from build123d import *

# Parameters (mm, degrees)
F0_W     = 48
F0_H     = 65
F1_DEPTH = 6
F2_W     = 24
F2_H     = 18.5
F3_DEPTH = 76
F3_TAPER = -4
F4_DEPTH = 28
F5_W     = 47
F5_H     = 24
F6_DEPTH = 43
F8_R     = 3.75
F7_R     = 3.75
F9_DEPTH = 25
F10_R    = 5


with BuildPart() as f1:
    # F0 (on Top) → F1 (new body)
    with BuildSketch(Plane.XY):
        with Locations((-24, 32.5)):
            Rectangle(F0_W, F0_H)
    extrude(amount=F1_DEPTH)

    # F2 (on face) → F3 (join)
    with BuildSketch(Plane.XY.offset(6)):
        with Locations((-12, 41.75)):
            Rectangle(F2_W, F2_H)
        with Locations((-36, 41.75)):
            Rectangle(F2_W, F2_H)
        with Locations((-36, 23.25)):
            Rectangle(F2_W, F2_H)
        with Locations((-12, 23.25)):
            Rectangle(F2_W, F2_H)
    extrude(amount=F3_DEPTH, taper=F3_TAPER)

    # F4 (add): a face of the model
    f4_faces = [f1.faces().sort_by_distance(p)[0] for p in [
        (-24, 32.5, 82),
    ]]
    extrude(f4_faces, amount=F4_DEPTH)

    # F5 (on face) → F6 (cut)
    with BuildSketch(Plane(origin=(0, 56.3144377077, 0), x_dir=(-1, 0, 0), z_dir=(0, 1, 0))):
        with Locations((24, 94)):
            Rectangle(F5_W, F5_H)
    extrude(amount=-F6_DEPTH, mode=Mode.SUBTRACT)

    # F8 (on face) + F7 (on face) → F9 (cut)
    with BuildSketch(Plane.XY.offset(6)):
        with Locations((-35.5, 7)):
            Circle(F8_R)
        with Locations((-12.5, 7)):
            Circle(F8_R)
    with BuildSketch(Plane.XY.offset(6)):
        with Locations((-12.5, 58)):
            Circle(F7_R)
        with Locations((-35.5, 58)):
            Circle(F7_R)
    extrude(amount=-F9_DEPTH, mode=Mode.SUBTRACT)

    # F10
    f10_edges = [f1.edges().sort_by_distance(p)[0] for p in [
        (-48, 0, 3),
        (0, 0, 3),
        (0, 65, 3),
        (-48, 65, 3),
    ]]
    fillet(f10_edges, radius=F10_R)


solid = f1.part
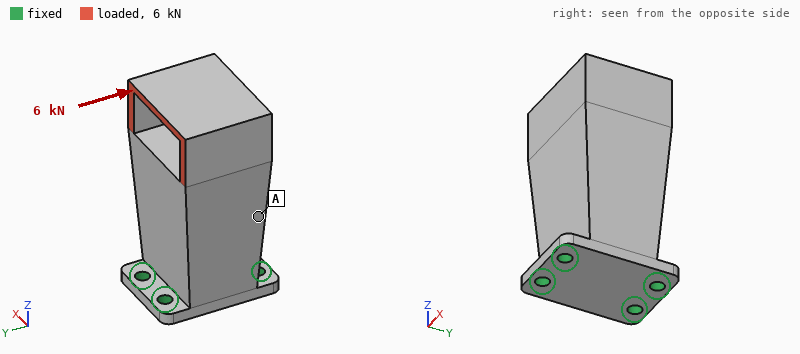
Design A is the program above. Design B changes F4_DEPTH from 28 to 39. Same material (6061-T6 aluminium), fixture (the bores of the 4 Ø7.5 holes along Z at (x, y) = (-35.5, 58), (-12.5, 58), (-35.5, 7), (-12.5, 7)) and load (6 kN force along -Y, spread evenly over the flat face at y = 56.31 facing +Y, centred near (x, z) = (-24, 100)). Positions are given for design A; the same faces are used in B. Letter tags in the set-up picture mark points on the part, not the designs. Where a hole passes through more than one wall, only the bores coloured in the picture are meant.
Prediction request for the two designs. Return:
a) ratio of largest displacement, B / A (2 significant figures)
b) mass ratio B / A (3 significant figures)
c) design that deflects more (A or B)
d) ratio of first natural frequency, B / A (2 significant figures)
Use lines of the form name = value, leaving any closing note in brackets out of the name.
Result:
ratio of largest displacement, B / A = 1.2
mass ratio B / A = 1.14
design that deflects more = B
ratio of first natural frequency, B / A = 0.80
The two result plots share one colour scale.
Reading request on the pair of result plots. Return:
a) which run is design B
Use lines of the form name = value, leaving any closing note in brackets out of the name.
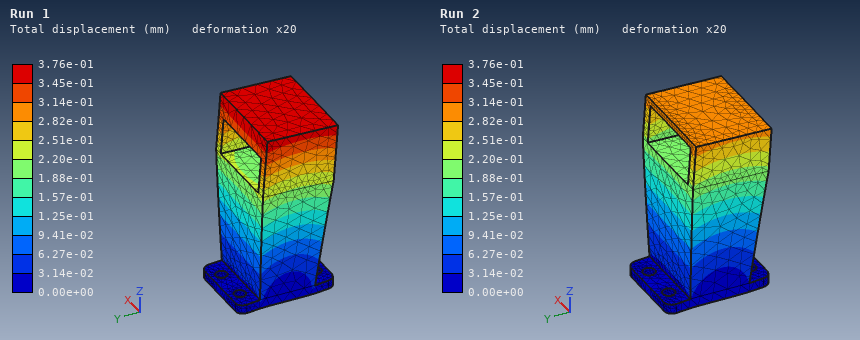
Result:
which run is design B = Run 1
